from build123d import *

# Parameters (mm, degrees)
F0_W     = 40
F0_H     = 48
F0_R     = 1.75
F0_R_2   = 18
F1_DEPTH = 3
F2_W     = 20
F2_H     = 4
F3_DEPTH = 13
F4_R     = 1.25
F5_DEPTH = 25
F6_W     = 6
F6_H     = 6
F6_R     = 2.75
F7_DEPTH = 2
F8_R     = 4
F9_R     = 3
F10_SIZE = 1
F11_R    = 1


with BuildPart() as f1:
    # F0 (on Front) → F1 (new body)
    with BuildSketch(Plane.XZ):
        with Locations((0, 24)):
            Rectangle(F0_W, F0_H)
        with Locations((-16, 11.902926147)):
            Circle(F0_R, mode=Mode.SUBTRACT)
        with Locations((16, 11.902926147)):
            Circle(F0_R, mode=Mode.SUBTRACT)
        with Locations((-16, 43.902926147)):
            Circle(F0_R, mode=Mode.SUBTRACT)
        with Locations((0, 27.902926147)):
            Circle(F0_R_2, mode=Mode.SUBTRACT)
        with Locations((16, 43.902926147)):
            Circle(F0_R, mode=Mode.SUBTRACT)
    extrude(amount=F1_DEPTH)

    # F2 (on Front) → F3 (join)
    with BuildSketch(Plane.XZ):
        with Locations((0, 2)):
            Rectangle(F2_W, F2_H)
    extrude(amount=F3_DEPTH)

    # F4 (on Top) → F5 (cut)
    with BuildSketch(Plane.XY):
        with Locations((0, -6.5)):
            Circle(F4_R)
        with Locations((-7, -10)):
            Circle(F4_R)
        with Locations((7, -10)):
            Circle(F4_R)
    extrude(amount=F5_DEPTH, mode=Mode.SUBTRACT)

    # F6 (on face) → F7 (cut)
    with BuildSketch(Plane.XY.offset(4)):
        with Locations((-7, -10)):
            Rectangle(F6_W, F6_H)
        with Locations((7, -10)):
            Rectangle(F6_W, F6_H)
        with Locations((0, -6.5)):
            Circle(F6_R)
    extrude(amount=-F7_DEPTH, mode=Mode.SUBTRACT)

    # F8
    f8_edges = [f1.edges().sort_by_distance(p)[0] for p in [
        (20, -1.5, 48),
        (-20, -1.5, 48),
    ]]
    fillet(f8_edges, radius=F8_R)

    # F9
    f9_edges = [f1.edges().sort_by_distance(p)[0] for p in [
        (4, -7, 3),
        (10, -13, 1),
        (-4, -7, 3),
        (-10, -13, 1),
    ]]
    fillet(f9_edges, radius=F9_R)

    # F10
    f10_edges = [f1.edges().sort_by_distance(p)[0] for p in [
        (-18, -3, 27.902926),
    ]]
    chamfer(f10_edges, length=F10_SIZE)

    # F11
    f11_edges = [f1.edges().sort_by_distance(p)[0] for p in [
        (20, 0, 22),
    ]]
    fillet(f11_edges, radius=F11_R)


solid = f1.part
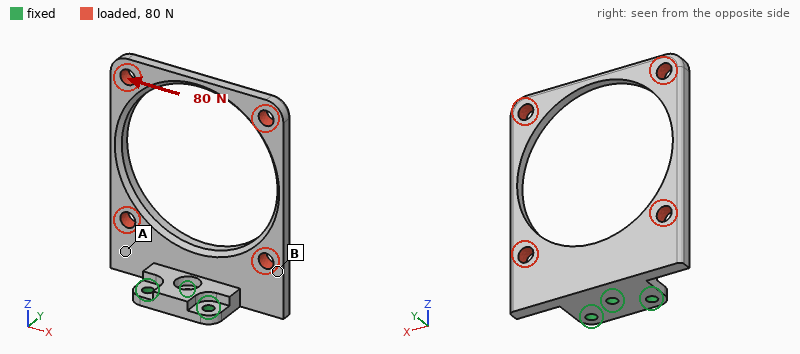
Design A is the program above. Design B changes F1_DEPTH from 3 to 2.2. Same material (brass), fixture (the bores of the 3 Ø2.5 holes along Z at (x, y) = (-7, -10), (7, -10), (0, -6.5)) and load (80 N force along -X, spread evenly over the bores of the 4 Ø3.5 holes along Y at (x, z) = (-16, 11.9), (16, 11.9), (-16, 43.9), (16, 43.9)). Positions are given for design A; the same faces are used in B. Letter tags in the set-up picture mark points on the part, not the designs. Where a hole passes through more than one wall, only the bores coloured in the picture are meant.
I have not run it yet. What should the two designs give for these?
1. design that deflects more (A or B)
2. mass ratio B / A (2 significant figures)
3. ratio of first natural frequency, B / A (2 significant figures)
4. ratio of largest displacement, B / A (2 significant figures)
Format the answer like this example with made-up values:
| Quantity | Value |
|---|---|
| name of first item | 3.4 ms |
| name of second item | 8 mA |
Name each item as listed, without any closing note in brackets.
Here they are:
| Quantity | Value |
|---|---|
| design that deflects more | B |
| mass ratio B / A | 0.80 |
| ratio of first natural frequency, B / A | 0.77 |
| ratio of largest displacement, B / A | 1.4 |
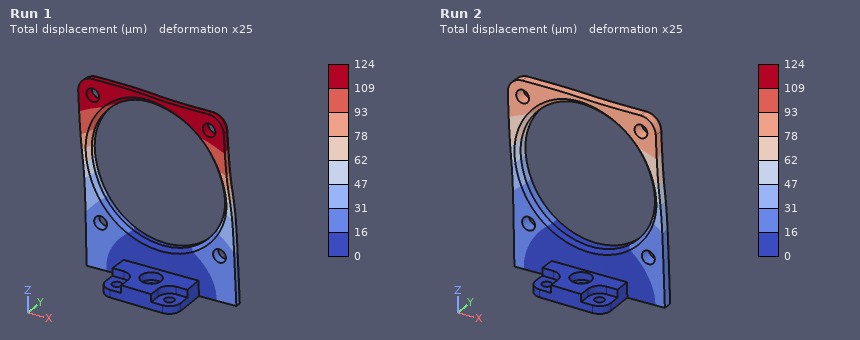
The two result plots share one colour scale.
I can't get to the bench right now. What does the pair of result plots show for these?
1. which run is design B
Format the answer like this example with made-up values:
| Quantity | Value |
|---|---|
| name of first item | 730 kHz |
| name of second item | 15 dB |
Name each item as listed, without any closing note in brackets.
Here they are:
| Quantity | Value |
|---|---|
| which run is design B | Run 1 |
